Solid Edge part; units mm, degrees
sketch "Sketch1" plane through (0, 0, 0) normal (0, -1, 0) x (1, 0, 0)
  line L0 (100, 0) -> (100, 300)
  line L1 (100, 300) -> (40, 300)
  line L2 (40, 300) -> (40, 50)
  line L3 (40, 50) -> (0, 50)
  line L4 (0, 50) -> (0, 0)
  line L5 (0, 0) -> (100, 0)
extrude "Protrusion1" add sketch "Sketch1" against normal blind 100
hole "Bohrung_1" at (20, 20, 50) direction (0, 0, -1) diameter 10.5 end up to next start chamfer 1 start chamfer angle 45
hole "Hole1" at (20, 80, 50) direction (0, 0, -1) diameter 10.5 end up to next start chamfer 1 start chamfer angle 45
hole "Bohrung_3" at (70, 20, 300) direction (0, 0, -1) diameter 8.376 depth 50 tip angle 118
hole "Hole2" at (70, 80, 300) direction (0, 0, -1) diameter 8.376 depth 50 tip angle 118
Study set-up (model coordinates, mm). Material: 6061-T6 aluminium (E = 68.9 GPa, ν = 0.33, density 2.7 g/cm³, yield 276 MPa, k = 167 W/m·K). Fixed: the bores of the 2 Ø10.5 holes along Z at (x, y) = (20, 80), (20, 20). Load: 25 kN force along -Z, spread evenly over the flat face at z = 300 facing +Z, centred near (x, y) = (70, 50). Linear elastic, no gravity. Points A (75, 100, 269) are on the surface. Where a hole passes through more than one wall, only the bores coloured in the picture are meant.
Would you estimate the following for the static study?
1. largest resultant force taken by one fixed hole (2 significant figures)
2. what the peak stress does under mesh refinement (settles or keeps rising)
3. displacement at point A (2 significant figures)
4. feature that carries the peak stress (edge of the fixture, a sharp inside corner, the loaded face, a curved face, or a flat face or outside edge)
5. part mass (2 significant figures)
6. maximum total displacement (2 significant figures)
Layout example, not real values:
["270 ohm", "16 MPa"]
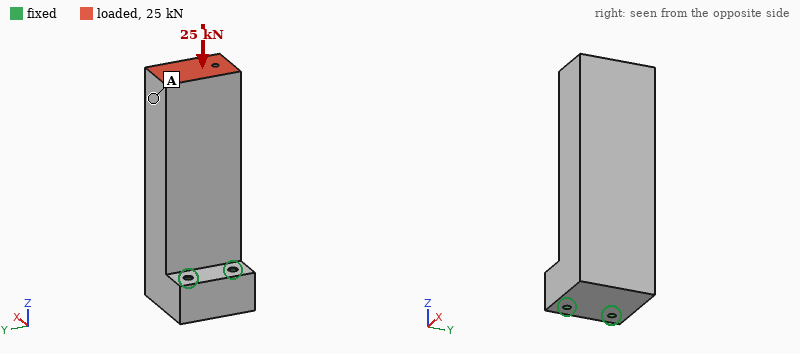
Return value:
["13 kN", "keeps rising", "0.16 mm", "edge of the fixture", "5.4 kg", "0.19 mm"]
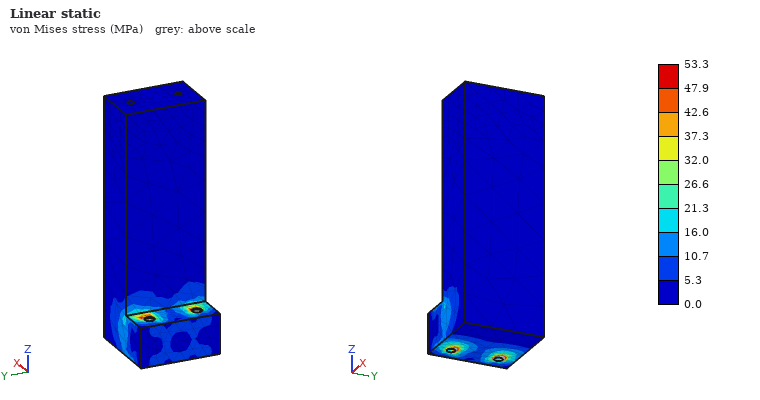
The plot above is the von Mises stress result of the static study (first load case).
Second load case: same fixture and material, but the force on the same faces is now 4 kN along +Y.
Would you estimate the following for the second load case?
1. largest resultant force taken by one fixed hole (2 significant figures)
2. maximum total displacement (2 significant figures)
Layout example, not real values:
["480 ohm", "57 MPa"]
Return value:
["13 kN", "0.18 mm"]
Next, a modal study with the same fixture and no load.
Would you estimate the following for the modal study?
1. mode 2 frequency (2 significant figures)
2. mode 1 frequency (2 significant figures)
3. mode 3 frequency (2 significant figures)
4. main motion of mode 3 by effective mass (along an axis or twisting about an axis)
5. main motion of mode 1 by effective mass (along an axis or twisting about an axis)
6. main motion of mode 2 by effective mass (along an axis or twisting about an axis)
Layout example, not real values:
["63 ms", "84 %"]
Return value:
["660 Hz", "440 Hz", "2200 Hz", "twisting about Z", "along X", "along Y"]
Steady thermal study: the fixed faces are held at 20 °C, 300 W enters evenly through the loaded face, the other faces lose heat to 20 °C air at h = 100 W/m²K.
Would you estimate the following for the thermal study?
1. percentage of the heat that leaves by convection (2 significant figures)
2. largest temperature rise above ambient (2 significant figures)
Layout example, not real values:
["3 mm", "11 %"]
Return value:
["68 %", "49 K"]
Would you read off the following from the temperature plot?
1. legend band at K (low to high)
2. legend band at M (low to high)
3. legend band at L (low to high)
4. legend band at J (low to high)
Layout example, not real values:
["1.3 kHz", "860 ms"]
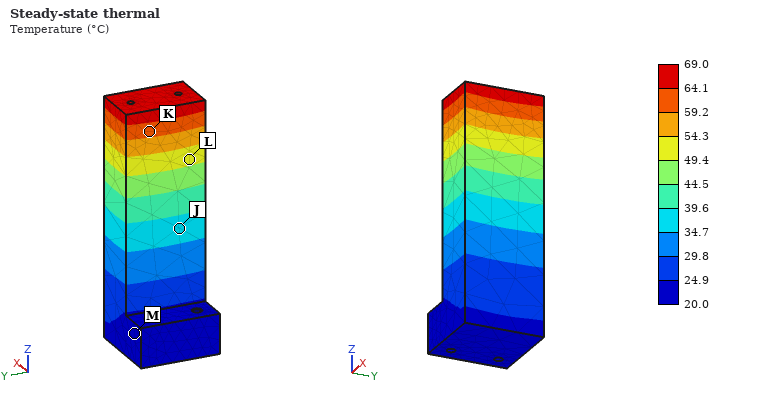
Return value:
["59.2 to 64.1 °C", "20.0 to 24.9 °C", "49.4 to 54.3 °C", "34.7 to 39.6 °C"]
